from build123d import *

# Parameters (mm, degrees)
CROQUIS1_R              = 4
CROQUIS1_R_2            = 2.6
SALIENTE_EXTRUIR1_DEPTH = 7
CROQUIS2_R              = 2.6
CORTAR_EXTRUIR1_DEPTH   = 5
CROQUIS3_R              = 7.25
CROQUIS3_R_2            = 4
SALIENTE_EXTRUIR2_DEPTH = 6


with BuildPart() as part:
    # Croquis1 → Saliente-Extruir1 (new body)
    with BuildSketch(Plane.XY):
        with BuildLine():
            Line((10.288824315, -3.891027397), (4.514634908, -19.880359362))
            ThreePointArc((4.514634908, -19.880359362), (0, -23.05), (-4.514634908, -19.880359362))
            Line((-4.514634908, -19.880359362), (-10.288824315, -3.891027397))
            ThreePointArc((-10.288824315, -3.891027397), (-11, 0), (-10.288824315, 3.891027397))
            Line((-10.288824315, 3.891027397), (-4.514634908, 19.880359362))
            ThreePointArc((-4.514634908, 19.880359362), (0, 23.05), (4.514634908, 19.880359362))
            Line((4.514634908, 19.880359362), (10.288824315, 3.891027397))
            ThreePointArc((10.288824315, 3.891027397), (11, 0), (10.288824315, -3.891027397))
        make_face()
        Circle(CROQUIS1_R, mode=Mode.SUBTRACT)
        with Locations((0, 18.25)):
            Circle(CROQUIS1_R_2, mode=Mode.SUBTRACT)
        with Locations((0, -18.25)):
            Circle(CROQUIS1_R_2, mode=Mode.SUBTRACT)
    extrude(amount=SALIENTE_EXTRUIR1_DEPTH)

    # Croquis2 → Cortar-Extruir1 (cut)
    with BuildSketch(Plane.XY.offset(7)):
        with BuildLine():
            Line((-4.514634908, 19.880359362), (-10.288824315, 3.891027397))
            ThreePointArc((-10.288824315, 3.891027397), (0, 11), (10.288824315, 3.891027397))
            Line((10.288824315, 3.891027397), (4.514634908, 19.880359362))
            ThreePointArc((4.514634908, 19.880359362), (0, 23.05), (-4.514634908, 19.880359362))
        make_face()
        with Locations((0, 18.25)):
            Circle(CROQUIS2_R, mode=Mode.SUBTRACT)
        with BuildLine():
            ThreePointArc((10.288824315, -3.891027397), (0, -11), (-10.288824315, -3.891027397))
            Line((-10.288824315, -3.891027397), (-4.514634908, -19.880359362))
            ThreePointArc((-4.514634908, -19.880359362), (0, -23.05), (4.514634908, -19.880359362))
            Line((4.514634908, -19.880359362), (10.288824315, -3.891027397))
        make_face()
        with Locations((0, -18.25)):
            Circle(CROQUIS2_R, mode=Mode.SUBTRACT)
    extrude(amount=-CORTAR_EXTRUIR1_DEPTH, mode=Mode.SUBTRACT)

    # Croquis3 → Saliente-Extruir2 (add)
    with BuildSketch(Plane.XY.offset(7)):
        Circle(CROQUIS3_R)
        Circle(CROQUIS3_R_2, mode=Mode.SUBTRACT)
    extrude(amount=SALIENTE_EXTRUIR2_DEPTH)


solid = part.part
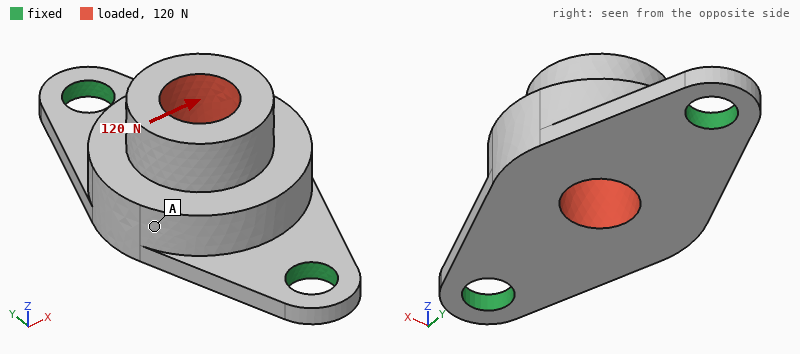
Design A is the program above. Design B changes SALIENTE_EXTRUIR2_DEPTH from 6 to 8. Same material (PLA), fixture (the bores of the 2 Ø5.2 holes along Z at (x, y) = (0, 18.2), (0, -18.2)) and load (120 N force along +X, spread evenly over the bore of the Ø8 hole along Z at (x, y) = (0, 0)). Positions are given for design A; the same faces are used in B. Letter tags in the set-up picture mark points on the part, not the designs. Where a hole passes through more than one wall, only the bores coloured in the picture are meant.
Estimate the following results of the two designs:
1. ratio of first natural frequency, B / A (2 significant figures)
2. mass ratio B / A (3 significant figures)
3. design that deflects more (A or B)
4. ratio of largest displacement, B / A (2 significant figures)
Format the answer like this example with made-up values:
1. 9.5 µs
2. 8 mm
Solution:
1. 0.90
2. 1.07
3. B
4. 1.3
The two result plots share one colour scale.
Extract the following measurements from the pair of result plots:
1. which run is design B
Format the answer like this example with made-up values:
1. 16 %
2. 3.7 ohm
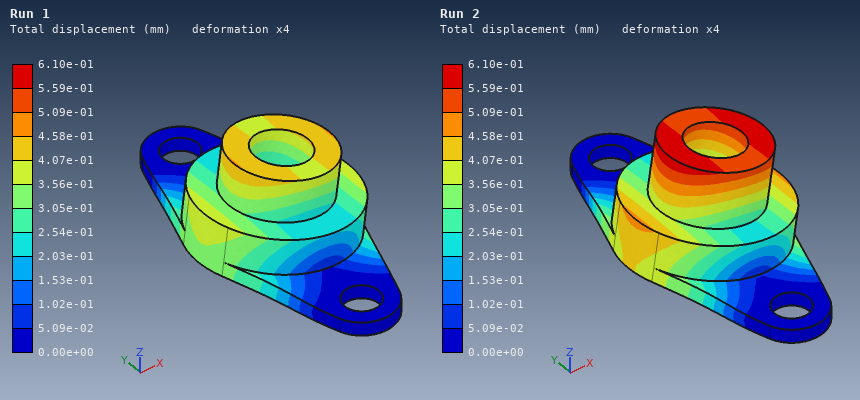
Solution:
1. Run 2
